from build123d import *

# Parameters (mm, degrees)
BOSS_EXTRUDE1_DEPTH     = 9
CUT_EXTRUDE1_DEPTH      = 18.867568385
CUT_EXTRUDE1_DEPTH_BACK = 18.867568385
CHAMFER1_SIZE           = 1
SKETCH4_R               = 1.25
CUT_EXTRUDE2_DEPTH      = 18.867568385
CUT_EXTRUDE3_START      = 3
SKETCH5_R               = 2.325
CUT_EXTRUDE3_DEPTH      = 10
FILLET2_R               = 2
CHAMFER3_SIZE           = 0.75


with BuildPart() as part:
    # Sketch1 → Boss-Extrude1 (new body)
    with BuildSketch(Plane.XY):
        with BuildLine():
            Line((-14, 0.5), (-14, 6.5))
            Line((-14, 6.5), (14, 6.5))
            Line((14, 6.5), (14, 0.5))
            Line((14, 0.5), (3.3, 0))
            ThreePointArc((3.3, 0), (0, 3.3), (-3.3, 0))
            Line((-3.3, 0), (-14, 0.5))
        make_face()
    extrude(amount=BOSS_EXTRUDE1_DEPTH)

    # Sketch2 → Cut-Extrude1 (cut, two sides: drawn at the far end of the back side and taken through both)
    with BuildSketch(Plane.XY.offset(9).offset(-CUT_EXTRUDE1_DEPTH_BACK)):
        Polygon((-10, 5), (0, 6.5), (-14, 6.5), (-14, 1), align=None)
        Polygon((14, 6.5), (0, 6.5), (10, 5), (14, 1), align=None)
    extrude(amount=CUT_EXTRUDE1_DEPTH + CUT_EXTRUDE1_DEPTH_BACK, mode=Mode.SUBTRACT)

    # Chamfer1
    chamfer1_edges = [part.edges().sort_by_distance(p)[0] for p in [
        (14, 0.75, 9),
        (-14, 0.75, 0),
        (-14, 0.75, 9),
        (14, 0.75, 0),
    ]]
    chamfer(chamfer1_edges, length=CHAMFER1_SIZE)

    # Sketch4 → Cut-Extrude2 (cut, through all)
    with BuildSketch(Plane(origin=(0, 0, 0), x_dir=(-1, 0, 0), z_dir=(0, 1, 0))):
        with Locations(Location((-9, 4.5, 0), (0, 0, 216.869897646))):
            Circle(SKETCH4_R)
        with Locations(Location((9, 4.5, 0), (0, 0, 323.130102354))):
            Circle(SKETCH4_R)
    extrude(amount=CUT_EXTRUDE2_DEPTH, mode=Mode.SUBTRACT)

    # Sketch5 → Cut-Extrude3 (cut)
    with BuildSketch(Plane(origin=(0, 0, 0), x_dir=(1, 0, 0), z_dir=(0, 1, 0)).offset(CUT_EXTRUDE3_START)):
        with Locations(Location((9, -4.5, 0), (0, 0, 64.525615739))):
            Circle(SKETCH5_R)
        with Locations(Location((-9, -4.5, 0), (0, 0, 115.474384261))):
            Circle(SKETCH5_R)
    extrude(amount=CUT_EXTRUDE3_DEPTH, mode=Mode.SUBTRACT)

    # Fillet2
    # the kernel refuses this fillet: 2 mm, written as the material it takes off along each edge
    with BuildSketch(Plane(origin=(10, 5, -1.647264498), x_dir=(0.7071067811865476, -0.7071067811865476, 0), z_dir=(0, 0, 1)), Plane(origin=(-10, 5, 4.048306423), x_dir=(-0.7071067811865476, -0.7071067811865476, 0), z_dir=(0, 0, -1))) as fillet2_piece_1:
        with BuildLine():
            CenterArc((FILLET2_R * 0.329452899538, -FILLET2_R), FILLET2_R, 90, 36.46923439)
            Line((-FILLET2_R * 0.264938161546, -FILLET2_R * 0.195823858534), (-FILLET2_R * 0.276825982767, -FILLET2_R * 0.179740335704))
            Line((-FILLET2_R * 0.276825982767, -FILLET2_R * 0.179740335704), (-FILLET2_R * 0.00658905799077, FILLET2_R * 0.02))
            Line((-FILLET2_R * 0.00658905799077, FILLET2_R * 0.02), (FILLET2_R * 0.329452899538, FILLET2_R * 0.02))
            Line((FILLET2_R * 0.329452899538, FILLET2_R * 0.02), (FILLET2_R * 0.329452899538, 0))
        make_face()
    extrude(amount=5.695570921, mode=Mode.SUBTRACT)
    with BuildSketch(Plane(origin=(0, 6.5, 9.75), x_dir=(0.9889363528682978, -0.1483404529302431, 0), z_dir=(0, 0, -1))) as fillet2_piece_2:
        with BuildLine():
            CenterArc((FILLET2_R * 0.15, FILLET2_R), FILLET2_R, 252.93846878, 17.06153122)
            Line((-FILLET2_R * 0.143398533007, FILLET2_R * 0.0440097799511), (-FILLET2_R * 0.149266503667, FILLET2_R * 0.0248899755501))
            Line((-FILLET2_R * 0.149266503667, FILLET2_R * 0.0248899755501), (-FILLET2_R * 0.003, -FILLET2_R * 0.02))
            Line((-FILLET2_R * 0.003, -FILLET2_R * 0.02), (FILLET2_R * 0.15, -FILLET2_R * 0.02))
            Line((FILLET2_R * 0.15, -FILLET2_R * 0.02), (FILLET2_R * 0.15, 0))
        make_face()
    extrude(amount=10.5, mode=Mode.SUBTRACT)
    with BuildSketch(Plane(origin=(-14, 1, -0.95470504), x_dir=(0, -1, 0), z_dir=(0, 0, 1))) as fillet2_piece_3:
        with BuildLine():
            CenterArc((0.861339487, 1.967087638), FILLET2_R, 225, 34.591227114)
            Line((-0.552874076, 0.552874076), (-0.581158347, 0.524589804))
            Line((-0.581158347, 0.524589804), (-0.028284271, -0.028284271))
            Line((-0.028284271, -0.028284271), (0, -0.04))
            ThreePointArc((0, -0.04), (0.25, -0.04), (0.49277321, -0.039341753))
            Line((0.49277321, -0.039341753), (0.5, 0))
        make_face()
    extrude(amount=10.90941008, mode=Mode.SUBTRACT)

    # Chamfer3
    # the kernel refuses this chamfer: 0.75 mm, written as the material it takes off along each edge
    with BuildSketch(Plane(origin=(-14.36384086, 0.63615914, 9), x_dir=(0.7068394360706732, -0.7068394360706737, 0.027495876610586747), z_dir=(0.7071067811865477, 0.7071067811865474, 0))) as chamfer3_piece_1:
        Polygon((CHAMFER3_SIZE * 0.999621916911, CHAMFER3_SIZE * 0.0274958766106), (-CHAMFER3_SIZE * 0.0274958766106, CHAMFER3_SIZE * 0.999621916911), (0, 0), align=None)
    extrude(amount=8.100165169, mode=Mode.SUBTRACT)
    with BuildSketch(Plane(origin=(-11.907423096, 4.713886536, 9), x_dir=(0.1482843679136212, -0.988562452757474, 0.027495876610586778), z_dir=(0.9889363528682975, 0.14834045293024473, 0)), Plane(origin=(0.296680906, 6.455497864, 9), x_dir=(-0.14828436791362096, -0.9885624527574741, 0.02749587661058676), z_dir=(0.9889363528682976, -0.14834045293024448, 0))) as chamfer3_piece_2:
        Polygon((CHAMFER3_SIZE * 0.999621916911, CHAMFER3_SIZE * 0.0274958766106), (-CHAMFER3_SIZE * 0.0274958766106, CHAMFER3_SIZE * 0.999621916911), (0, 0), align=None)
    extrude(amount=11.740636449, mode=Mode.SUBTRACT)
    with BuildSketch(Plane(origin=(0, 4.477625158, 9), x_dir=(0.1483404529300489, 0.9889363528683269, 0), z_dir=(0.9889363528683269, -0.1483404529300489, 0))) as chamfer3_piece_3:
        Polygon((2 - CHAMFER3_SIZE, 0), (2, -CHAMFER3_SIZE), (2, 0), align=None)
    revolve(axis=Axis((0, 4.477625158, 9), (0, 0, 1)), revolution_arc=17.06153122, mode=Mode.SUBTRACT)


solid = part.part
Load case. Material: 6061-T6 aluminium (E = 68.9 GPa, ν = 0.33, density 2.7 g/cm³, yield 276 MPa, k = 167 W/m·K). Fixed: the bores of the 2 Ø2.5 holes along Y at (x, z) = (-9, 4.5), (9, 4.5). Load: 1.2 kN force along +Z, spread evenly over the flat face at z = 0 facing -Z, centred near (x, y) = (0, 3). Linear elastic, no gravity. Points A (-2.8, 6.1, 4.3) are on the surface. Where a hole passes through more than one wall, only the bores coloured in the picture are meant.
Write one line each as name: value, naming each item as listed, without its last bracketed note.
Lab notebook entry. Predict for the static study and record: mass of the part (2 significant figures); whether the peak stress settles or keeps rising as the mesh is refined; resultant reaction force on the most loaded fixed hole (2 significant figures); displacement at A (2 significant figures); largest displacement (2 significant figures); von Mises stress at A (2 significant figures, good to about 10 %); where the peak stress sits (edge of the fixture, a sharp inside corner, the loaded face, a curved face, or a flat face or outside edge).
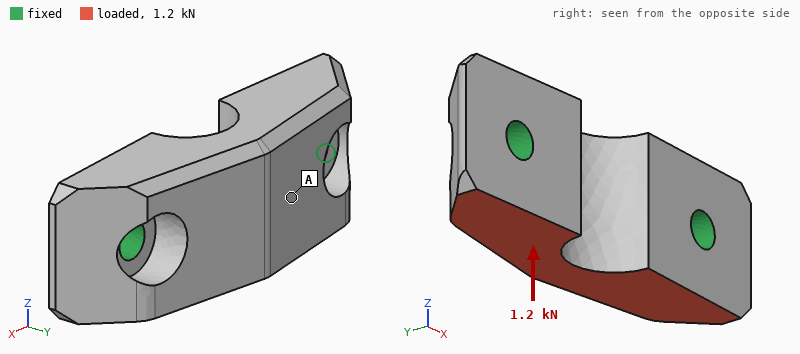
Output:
mass of the part: 2.5 g
whether the peak stress settles or keeps rising as the mesh is refined: keeps rising
resultant reaction force on the most loaded fixed hole: 600 N
displacement at A: 9.3 µm
largest displacement: 13 µm
von Mises stress at A: 20 MPa
where the peak stress sits: edge of the fixture
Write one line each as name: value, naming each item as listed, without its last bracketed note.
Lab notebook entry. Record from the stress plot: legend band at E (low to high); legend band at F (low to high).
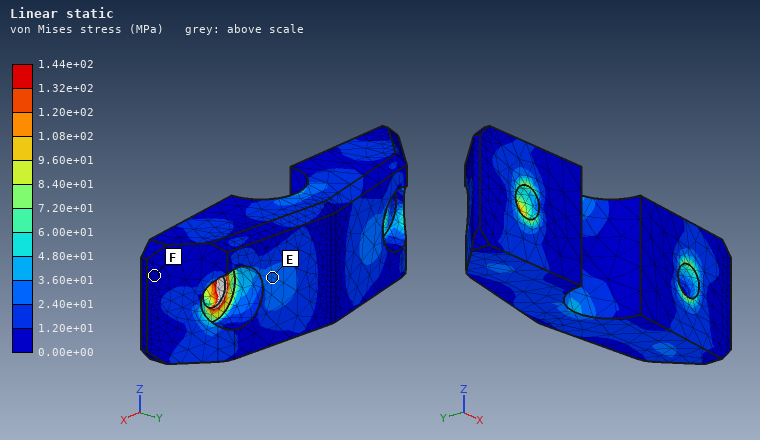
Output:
legend band at E: 2.40e+01 to 3.60e+01 MPa
legend band at F: 0.00e+00 to 1.20e+01 MPa
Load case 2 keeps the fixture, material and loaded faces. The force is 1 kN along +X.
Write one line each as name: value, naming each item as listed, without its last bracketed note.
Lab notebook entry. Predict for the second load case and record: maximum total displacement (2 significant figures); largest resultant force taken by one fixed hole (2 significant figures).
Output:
maximum total displacement: 4.7 µm
largest resultant force taken by one fixed hole: 540 N
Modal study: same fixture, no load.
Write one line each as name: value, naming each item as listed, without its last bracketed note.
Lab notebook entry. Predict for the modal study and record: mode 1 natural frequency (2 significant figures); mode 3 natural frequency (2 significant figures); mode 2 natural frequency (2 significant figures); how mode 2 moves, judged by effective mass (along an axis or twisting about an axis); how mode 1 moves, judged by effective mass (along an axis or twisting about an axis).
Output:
mode 1 natural frequency: 36 kHz
mode 3 natural frequency: 65 kHz
mode 2 natural frequency: 51 kHz
how mode 2 moves, judged by effective mass: along Y
how mode 1 moves, judged by effective mass: along Z
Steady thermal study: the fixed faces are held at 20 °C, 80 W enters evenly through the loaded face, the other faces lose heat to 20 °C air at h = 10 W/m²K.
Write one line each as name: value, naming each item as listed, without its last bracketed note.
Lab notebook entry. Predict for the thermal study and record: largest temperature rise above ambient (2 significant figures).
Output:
largest temperature rise above ambient: 40 K
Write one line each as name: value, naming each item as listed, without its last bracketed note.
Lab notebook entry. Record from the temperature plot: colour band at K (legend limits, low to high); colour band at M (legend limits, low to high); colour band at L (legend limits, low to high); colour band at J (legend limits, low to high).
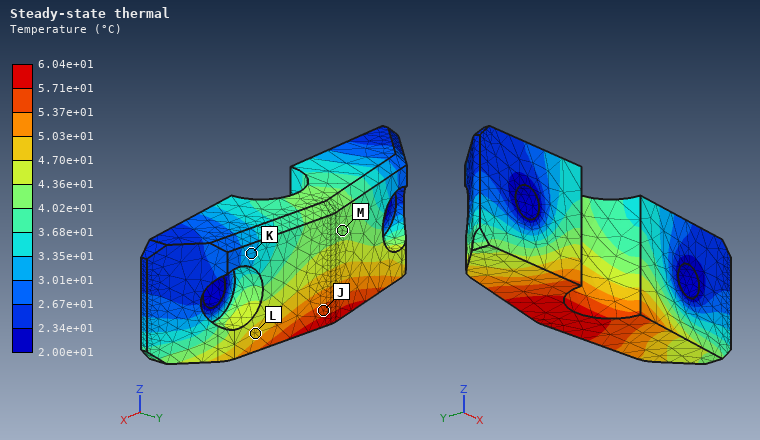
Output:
colour band at K: 3.01e+01 to 3.35e+01 °C
colour band at M: 4.02e+01 to 4.36e+01 °C
colour band at L: 4.70e+01 to 5.03e+01 °C
colour band at J: 5.37e+01 to 5.71e+01 °C
